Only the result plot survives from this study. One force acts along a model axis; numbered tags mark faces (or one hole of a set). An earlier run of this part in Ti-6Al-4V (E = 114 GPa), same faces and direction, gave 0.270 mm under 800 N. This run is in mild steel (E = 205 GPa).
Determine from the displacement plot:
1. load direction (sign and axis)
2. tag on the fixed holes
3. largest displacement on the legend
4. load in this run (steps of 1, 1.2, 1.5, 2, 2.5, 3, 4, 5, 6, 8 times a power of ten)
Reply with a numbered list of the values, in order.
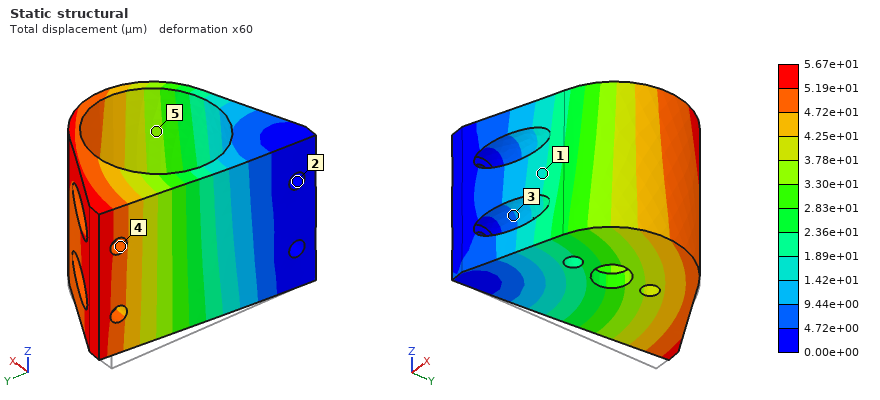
1. +X
2. 2
3. 5.67e+01 µm
4. 300 N
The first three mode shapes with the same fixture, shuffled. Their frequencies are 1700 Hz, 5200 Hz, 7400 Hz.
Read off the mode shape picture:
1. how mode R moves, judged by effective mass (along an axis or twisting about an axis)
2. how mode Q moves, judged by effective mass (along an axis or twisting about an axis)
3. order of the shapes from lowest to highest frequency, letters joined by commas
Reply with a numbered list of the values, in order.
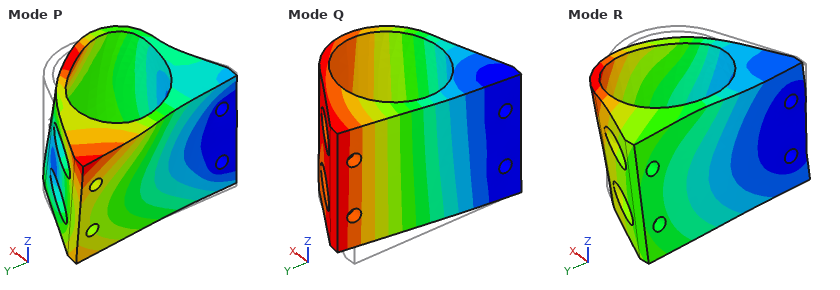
1. along Z
2. along X
3. Q, R, P
